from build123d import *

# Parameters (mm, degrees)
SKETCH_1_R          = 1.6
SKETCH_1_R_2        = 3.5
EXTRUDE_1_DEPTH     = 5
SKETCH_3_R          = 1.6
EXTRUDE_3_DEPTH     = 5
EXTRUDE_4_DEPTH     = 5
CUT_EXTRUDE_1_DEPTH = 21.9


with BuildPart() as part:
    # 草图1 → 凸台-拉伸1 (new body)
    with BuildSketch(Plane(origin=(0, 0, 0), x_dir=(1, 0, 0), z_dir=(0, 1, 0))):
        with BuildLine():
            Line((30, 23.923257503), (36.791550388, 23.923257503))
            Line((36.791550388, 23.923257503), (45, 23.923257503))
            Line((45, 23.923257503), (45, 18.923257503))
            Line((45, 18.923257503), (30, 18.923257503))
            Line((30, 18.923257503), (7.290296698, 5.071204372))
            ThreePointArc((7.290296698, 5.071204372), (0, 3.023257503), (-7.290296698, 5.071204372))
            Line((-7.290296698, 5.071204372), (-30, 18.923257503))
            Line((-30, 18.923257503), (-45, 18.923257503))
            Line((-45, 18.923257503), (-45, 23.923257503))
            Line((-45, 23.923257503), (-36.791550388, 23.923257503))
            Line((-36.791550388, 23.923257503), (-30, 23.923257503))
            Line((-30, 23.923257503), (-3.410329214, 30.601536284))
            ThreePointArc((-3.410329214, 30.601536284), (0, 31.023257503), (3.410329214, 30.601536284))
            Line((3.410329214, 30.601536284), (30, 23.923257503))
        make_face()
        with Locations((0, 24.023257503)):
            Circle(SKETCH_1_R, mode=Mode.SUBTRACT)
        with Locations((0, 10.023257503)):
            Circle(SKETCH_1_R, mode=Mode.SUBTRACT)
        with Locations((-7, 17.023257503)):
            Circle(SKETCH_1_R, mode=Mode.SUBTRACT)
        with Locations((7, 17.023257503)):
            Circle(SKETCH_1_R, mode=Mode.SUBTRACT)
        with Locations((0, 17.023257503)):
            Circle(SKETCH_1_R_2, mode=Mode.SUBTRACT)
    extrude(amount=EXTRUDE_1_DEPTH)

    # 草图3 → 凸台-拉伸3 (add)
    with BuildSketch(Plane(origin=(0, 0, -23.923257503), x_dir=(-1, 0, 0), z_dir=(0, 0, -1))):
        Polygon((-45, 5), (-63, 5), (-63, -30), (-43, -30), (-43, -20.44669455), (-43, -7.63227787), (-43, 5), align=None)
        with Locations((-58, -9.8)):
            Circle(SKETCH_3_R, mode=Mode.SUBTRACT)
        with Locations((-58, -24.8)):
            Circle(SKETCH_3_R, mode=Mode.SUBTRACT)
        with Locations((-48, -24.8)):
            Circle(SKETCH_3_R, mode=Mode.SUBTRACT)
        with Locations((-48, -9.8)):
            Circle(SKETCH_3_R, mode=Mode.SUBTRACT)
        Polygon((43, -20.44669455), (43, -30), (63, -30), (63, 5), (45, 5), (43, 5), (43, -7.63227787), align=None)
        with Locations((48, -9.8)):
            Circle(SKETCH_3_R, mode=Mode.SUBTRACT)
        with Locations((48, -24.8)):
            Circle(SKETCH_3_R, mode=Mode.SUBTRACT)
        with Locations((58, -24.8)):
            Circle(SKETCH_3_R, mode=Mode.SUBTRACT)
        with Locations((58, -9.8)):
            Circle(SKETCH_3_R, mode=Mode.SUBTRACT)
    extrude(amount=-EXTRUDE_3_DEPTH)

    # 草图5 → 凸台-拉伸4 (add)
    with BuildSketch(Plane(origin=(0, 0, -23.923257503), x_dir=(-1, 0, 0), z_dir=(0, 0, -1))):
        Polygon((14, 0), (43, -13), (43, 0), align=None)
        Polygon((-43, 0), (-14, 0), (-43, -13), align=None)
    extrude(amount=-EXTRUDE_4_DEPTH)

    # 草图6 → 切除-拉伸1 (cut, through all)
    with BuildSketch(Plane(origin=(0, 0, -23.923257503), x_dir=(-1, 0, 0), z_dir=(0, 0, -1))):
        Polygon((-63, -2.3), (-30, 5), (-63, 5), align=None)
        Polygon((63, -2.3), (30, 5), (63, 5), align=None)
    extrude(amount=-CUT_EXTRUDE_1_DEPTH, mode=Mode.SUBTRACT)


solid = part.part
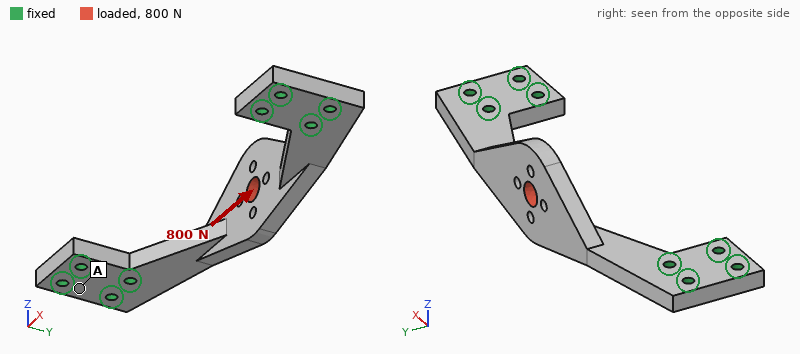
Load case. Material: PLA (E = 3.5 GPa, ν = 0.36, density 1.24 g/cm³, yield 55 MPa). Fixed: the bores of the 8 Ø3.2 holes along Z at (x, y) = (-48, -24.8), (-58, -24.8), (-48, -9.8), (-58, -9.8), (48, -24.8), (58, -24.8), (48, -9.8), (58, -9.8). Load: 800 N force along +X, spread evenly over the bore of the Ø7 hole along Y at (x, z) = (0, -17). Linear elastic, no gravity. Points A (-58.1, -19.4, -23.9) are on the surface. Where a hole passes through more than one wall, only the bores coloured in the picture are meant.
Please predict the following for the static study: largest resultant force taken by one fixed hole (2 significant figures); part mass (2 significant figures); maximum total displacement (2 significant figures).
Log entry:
290 N
16 g
0.26 mm
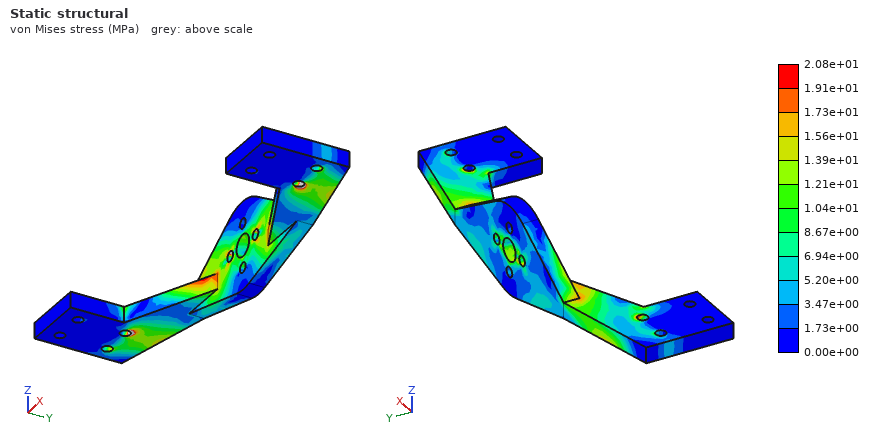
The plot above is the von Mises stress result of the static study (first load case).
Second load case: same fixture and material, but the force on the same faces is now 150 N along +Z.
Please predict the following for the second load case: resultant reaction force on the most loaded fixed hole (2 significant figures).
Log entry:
120 N
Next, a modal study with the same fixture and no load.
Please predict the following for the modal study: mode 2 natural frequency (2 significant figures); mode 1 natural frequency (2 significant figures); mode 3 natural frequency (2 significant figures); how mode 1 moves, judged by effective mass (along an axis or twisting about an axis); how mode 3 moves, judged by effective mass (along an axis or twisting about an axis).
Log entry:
1600 Hz
1000 Hz
2400 Hz
along Z
along Y
